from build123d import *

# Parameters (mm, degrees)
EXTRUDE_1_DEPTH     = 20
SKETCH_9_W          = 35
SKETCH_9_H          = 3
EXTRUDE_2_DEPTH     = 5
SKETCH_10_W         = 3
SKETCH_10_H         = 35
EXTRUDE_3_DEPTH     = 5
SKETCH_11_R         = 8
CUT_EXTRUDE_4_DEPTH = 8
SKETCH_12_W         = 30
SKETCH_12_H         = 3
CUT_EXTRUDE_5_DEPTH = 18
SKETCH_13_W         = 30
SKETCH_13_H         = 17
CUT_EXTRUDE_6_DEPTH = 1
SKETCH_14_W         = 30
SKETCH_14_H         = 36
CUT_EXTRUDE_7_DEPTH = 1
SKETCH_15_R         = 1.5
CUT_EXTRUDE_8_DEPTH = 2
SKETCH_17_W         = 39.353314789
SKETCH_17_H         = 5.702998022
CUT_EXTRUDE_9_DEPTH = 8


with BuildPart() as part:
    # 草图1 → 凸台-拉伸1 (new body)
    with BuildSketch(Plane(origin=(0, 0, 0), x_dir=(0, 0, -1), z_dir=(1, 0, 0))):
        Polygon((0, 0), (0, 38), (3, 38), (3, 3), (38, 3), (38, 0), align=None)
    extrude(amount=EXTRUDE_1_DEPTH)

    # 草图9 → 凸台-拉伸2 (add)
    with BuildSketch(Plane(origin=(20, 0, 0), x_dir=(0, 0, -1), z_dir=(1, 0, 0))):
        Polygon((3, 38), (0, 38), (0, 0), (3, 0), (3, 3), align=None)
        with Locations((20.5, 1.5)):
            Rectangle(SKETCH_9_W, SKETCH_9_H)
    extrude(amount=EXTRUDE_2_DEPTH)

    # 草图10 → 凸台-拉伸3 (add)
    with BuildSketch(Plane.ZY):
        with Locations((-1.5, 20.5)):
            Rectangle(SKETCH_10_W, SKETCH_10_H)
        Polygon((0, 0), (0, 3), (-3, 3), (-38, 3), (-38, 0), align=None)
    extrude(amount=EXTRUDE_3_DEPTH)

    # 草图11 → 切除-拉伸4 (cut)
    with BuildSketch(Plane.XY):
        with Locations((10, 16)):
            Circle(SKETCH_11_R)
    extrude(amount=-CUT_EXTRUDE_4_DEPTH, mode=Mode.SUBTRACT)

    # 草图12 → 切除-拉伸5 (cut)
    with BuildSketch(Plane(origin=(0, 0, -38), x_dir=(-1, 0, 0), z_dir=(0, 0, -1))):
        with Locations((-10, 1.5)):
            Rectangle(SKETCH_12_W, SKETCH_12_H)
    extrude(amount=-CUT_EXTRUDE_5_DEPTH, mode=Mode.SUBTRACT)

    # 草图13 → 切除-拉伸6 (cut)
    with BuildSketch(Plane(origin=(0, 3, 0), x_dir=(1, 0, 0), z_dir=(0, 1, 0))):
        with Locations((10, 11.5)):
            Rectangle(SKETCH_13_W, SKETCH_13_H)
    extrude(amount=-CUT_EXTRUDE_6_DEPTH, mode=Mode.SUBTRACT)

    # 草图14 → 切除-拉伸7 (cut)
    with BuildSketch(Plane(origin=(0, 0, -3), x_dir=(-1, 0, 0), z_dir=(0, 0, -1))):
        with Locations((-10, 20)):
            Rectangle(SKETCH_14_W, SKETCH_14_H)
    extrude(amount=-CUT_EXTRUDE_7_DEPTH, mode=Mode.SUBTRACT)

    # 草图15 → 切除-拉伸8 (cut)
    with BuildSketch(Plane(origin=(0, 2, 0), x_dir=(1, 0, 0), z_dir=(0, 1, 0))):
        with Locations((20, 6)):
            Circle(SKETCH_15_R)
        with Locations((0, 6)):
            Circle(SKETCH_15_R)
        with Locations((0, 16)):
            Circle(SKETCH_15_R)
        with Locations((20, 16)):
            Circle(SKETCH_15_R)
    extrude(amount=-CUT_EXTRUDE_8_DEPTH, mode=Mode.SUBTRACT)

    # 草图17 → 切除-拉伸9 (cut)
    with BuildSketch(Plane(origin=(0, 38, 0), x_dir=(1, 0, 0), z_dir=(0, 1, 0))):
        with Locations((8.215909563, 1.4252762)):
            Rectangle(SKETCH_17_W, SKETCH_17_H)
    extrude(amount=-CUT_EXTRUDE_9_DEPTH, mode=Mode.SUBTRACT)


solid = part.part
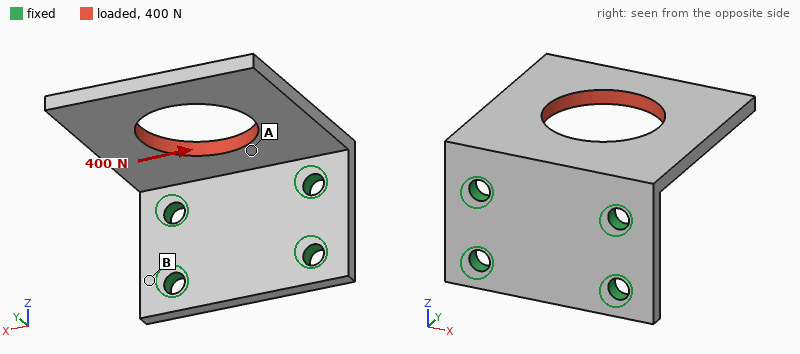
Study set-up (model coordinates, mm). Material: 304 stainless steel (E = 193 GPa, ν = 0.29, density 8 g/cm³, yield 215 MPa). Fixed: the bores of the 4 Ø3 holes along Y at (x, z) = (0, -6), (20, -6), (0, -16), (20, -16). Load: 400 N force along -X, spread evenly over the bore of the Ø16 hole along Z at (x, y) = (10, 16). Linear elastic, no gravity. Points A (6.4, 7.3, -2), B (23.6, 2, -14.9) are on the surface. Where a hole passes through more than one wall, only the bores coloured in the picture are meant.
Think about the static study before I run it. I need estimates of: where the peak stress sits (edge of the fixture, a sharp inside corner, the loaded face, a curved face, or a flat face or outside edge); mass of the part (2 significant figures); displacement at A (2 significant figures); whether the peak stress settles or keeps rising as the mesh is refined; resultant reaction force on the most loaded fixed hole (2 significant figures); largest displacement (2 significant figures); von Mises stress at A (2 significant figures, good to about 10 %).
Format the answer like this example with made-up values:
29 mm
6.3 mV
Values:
edge of the fixture
19 g
5.2 µm
keeps rising
350 N
29 µm
42 MPa
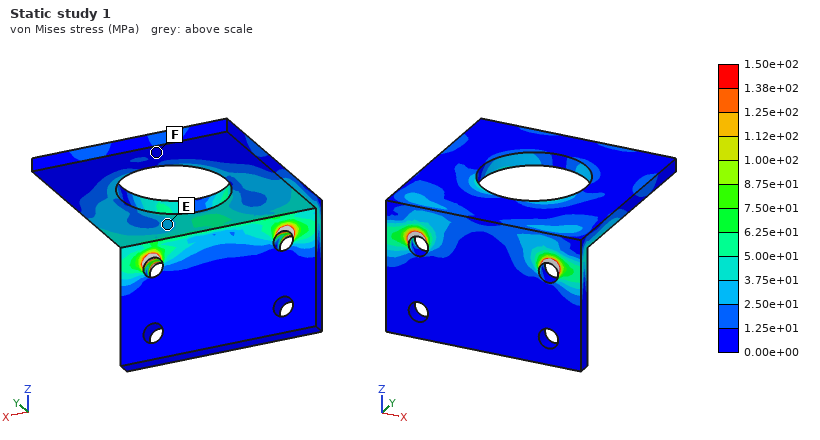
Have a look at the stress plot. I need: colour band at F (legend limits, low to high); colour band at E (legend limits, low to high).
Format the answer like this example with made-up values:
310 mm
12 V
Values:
0.00e+00 to 1.25e+01 MPa
2.50e+01 to 3.75e+01 MPa
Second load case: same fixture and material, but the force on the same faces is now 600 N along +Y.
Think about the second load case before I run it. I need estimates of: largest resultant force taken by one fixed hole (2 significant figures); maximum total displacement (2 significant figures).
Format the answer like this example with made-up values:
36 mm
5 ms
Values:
330 N
52 µm
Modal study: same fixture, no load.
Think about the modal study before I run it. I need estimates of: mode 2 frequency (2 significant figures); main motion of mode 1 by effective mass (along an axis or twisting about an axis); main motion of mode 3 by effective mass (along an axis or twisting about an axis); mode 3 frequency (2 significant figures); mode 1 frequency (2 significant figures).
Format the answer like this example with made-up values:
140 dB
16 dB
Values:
3500 Hz
along Z
along X
7500 Hz
1500 Hz
